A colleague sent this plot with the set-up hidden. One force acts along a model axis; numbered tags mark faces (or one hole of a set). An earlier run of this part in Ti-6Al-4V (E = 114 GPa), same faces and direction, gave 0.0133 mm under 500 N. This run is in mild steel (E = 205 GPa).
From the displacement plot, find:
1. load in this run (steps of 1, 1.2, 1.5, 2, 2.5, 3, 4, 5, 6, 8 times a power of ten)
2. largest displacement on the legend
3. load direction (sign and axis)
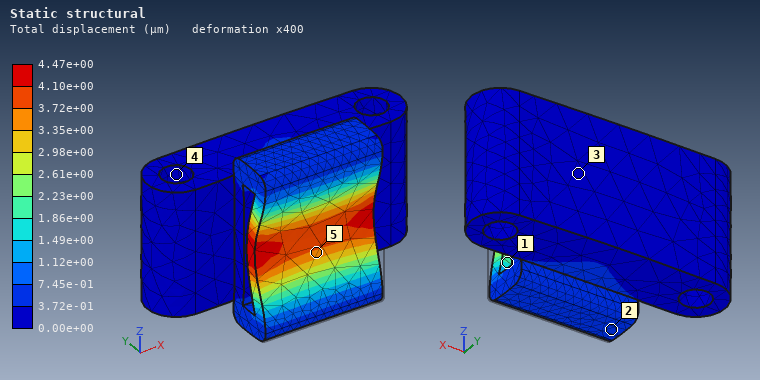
300 N
4.47e+00 µm
+Y
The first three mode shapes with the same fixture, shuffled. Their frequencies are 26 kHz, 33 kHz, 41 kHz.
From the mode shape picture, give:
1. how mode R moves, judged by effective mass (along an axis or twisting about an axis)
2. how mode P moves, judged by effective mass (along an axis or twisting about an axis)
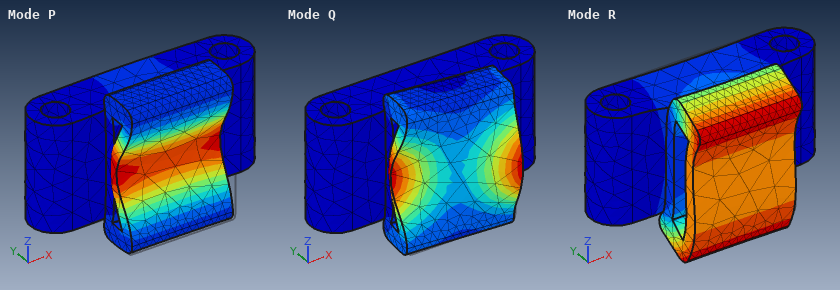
along Z
along Y
